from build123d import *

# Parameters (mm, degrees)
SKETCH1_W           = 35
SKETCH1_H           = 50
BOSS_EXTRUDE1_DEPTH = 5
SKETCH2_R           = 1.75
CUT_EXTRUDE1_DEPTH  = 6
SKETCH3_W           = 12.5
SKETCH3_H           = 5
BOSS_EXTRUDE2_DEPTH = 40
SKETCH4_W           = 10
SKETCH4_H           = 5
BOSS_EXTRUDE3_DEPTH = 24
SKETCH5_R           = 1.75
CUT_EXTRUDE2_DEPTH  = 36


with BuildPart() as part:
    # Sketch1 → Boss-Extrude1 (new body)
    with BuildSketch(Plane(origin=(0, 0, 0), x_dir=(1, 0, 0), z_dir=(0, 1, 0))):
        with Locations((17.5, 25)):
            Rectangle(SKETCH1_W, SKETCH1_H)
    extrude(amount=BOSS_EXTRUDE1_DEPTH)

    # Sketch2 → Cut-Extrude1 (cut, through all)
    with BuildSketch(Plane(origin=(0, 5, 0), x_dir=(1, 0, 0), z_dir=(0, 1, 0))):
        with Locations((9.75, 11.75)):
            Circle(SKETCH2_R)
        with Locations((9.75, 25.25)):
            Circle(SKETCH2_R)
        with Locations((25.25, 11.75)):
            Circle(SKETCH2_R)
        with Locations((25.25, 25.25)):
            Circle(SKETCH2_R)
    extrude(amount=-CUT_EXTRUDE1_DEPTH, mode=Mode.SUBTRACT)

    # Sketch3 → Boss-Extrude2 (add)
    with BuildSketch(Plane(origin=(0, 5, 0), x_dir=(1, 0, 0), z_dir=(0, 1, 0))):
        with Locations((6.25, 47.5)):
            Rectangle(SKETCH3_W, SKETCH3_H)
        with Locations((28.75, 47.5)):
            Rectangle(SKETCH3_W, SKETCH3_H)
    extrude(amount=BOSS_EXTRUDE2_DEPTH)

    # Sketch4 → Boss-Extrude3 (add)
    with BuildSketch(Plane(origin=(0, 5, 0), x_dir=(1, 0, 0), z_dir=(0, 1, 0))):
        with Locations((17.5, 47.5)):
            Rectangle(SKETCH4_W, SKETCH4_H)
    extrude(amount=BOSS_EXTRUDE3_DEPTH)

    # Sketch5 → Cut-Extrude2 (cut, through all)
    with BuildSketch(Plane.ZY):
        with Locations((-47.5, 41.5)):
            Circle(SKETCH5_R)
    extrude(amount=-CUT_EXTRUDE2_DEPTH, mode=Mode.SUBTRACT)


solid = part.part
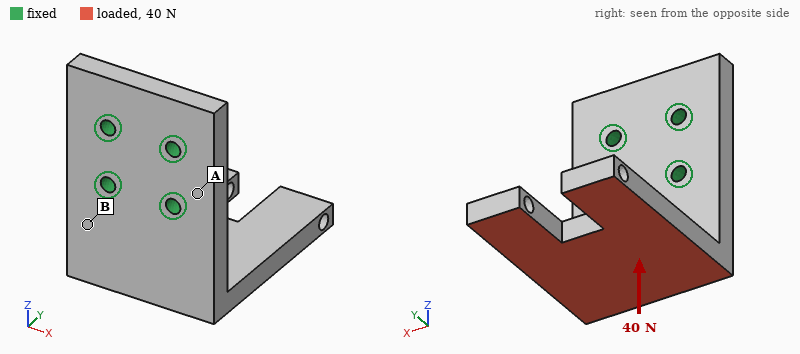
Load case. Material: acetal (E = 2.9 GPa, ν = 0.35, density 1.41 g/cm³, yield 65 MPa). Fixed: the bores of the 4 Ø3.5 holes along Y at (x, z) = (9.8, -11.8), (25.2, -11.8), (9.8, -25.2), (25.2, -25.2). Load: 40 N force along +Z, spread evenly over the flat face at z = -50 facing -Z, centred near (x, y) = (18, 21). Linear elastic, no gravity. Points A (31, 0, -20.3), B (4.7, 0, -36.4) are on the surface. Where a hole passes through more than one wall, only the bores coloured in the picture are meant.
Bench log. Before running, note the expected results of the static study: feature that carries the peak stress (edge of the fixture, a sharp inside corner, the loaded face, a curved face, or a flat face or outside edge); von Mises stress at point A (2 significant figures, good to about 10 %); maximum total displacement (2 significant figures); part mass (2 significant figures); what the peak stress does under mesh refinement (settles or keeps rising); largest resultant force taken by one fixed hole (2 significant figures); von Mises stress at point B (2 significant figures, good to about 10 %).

edge of the fixture
0.85 MPa
0.89 mm
20 g
keeps rising
19 N
4.6 MPa
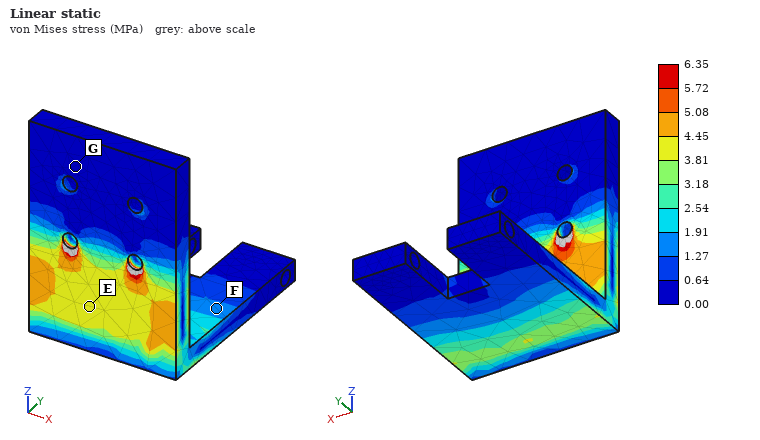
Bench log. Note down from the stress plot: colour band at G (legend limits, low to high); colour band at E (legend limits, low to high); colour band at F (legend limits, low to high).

0.00 to 0.64 MPa
3.81 to 4.45 MPa
1.27 to 1.91 MPa
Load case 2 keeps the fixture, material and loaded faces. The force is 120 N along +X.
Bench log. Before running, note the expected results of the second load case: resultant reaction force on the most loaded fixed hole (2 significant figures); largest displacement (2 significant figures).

170 N
0.87 mm
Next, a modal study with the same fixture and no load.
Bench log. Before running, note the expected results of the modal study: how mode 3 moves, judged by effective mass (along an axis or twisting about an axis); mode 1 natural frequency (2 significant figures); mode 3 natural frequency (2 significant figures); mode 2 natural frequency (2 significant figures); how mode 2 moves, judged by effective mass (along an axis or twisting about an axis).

along Y
420 Hz
1300 Hz
710 Hz
along X
